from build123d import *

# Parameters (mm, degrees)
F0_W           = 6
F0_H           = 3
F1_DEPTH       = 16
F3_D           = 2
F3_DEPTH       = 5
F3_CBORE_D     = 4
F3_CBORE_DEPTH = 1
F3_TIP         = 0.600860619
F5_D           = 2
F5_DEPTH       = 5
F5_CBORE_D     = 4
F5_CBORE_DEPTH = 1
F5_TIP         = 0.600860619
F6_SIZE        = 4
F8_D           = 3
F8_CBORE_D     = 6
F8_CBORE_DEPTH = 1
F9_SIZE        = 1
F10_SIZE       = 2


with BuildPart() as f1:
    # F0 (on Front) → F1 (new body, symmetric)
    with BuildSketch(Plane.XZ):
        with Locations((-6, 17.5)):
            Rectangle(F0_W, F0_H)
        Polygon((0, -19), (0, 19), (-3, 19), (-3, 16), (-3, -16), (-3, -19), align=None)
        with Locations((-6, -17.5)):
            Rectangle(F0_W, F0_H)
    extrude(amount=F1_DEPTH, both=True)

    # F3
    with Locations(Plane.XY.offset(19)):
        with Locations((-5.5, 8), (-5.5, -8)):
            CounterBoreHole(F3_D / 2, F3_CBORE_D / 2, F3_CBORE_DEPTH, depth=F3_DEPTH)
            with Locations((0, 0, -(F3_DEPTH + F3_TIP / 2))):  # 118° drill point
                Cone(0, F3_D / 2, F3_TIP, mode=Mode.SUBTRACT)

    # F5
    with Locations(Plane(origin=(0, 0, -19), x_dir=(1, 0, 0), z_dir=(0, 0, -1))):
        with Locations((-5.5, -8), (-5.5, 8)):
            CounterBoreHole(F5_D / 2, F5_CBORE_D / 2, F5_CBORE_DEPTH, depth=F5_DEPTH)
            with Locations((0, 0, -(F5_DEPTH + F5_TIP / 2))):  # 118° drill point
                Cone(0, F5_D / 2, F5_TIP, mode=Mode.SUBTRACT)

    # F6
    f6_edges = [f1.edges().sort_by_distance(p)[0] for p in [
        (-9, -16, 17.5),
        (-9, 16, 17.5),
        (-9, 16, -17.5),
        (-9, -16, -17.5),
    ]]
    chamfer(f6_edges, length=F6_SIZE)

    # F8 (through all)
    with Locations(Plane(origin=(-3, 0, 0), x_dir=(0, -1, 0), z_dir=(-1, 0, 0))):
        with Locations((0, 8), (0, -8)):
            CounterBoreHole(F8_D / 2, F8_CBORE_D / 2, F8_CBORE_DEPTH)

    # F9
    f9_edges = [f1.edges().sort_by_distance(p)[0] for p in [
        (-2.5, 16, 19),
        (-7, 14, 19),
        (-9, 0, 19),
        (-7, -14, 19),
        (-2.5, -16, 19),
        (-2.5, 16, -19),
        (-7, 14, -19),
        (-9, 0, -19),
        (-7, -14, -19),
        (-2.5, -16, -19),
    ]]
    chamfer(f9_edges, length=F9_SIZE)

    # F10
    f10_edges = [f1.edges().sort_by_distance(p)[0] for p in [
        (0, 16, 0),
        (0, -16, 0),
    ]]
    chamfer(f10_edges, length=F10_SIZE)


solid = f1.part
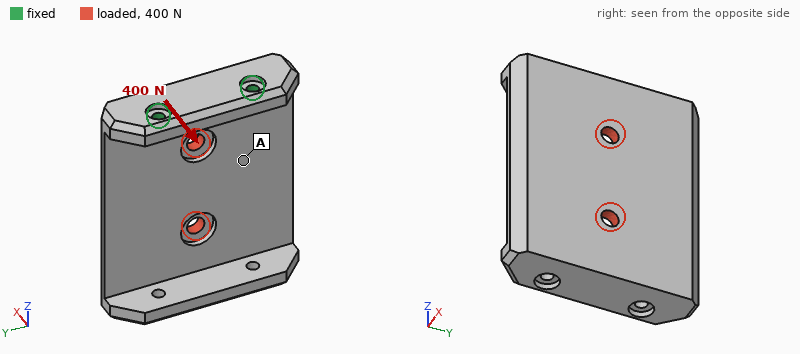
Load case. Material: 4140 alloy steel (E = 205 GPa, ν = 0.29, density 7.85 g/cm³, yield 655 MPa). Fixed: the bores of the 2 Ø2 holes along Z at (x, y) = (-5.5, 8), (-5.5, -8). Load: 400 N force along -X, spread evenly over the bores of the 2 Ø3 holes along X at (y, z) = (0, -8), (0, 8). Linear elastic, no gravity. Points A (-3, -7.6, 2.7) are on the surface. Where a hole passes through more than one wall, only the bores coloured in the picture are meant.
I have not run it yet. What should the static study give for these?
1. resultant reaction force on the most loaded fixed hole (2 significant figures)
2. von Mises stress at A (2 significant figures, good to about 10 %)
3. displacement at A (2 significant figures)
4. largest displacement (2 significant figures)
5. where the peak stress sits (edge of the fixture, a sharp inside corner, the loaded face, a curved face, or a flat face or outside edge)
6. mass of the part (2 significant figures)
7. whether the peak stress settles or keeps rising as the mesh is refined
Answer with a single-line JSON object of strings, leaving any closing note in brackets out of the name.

{"resultant reaction force on the most loaded fixed hole": "200 N", "von Mises stress at A": "48 MPa", "displacement at A": "0.097 mm", "largest displacement": "0.30 mm", "where the peak stress sits": "edge of the fixture", "mass of the part": "34 g", "whether the peak stress settles or keeps rising as the mesh is refined": "keeps rising"}
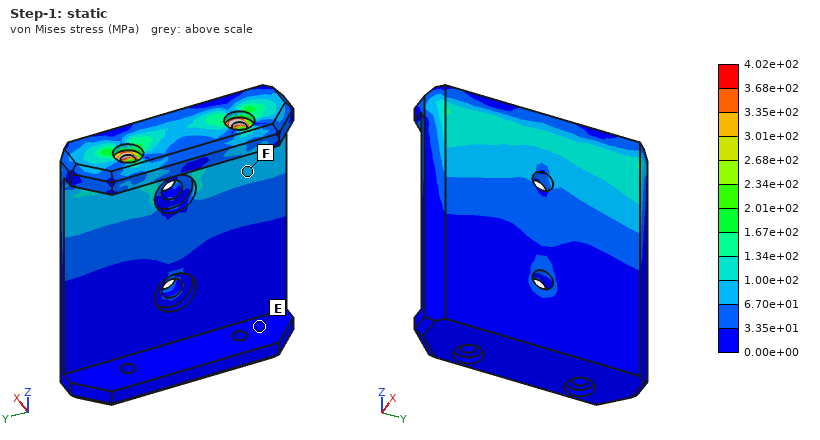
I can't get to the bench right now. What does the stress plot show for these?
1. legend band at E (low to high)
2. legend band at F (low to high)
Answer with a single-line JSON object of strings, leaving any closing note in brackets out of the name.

{"legend band at E": "0.00e+00 to 3.35e+01 MPa", "legend band at F": "6.70e+01 to 1.00e+02 MPa"}
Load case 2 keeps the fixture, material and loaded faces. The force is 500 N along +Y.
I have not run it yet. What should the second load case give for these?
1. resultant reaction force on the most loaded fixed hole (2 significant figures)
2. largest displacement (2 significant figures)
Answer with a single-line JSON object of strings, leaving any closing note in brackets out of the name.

{"resultant reaction force on the most loaded fixed hole": "560 N", "largest displacement": "23 µm"}
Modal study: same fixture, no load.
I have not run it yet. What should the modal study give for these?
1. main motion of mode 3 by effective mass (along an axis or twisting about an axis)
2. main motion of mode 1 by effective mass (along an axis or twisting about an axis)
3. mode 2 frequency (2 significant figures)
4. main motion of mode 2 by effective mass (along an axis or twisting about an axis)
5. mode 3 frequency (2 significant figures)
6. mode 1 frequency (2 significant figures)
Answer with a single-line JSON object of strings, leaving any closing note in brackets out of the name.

{"main motion of mode 3 by effective mass": "along Y", "main motion of mode 1 by effective mass": "along X", "mode 2 frequency": "3500 Hz", "main motion of mode 2 by effective mass": "along Y", "mode 3 frequency": "5400 Hz", "mode 1 frequency": "1100 Hz"}
